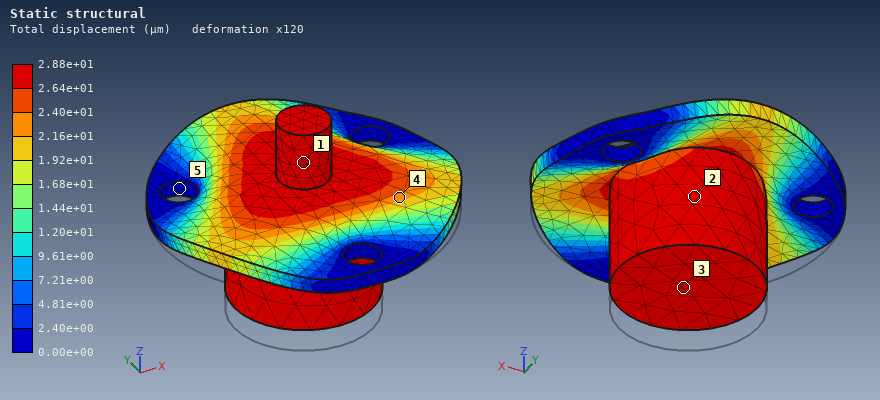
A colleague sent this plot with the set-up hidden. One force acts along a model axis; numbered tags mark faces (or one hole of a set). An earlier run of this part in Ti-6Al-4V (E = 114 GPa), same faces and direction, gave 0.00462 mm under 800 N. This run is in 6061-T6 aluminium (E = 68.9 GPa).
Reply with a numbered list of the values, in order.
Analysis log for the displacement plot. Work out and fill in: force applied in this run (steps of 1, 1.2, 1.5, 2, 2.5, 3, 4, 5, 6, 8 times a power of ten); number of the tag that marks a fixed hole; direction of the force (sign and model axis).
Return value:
1. 3 kN
2. 5
3. +Z
